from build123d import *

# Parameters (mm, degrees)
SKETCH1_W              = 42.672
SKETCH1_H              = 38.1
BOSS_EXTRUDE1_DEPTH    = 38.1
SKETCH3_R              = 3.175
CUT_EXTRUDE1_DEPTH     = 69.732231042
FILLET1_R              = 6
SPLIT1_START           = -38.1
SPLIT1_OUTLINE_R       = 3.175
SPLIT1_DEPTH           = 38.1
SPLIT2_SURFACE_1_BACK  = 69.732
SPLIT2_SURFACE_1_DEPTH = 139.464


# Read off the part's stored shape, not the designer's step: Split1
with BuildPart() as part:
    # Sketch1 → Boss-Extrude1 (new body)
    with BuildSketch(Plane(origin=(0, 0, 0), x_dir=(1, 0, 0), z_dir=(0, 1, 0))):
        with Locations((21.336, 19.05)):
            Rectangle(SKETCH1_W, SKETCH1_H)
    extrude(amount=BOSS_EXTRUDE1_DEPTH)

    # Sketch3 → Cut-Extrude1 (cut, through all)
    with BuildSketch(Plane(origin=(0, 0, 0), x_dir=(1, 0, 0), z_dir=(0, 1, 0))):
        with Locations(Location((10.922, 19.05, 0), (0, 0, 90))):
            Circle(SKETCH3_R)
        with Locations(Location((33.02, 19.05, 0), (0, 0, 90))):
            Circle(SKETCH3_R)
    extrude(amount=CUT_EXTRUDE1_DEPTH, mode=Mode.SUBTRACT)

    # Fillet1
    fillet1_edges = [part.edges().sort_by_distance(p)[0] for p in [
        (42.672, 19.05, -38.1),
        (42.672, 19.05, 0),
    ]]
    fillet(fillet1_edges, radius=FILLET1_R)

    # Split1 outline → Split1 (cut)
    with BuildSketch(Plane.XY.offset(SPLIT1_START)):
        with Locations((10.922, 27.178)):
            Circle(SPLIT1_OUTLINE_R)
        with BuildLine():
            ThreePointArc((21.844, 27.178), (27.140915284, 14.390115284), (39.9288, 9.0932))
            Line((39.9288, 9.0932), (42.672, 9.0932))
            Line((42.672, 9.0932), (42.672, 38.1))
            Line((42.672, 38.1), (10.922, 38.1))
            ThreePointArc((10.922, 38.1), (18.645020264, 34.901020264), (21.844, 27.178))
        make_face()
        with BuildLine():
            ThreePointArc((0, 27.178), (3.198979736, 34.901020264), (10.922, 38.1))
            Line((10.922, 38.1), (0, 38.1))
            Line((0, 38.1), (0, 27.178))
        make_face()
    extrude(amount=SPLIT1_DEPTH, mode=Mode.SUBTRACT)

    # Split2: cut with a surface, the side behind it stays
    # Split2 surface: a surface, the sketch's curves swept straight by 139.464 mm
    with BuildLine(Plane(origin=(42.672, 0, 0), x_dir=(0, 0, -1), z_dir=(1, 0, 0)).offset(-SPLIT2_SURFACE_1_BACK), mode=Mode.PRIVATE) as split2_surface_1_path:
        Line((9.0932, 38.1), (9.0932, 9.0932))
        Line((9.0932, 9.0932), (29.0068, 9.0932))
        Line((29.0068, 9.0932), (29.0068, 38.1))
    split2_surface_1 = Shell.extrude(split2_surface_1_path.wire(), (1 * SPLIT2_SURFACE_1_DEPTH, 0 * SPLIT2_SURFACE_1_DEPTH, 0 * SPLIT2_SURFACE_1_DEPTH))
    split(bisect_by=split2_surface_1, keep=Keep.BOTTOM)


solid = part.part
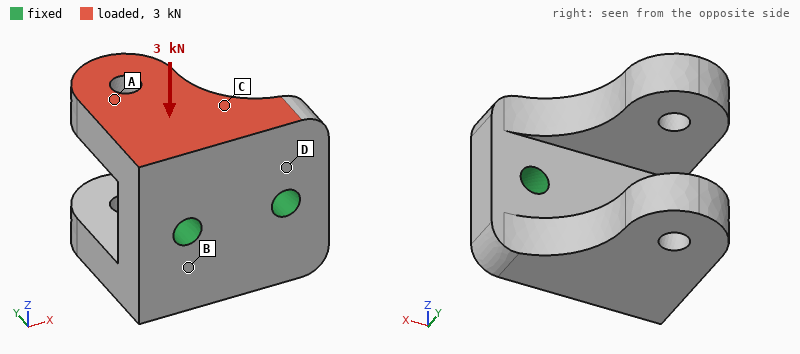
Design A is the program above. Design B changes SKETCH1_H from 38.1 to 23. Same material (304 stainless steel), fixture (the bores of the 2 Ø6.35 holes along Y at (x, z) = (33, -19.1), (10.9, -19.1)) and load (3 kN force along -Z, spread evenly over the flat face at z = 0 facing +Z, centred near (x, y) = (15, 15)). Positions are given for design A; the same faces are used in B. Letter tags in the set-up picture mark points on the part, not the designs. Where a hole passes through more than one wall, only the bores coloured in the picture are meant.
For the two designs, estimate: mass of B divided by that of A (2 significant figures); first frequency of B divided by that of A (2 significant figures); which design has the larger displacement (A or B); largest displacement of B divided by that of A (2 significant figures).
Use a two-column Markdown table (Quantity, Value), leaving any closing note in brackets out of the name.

| Quantity | Value |
|---|---|
| mass of B divided by that of A | 0.40 |
| first frequency of B divided by that of A | 0.34 |
| which design has the larger displacement | B |
| largest displacement of B divided by that of A | 60 |
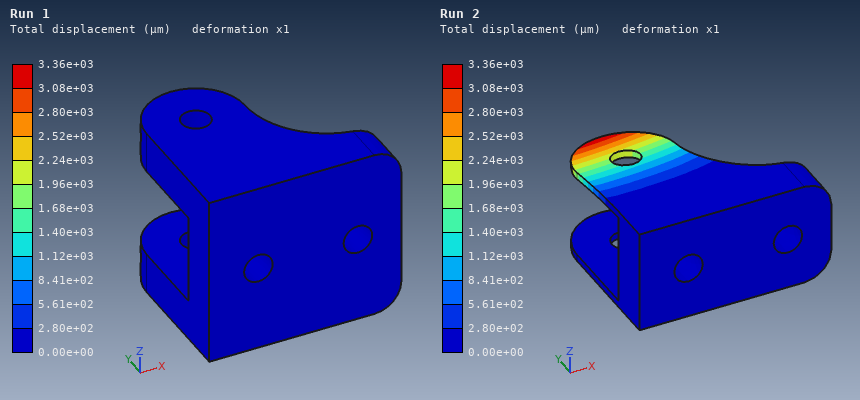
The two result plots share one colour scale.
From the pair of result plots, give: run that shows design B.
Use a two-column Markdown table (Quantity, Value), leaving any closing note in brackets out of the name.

| Quantity | Value |
|---|---|
| run that shows design B | Run 2 |
